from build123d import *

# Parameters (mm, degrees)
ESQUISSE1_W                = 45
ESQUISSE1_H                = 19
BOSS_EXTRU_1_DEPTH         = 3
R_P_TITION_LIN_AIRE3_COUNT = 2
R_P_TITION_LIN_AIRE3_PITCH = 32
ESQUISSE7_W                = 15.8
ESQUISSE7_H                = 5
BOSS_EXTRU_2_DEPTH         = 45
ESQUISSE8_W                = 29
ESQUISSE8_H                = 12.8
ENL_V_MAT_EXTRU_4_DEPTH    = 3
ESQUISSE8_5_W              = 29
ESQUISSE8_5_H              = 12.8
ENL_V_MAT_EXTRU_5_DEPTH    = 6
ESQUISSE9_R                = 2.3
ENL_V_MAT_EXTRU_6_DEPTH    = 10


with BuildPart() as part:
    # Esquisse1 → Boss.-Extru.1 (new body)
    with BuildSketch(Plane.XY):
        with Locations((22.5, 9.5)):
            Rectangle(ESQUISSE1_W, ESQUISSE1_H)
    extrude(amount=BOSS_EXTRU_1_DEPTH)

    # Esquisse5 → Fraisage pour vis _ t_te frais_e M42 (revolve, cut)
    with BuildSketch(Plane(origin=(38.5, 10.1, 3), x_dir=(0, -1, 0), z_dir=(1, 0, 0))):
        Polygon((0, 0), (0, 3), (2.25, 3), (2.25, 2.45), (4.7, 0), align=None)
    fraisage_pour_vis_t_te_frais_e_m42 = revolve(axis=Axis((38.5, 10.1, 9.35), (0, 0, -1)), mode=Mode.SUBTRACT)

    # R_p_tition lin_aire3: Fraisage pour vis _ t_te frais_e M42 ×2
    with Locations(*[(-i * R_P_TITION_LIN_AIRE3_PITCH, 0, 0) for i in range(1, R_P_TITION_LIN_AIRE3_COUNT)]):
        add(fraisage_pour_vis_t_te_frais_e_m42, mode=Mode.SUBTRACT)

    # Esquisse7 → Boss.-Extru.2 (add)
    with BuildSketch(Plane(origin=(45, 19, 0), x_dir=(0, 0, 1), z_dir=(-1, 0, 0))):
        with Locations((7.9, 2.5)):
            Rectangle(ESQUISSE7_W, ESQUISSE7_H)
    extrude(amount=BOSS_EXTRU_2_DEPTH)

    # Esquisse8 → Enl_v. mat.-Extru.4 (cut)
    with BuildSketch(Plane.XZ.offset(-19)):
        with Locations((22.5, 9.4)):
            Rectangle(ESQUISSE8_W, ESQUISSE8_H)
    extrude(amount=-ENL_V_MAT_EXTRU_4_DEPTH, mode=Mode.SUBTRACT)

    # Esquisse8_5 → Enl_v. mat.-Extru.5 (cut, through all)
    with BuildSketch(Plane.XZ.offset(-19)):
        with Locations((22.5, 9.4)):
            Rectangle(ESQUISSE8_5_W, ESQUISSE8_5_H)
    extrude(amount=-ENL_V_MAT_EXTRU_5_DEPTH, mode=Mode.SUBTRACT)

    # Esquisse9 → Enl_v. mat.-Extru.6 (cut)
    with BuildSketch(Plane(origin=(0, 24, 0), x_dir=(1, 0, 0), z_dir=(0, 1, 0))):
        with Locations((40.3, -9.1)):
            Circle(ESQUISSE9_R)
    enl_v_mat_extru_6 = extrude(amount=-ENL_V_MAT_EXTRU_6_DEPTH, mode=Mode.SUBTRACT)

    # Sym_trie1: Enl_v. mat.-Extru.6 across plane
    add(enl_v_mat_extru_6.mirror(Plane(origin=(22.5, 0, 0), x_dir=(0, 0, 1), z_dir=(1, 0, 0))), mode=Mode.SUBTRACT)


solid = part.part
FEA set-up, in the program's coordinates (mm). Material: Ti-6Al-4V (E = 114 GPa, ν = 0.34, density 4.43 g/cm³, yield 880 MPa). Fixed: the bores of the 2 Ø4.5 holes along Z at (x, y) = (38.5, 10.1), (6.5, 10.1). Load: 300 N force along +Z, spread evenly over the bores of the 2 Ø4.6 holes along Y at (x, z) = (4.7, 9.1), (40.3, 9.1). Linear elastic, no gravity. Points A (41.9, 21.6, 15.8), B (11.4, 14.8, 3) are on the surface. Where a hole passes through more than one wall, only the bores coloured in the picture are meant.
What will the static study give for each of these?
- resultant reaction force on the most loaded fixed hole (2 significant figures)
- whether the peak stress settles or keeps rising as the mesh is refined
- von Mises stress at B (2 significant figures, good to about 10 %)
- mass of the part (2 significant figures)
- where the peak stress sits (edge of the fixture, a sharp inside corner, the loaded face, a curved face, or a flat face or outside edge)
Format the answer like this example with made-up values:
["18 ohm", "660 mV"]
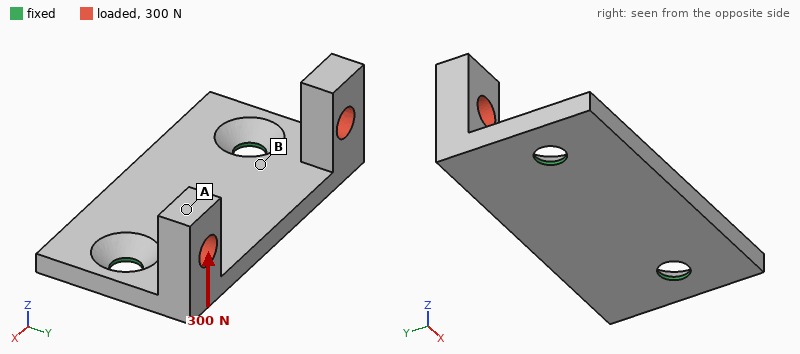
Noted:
["150 N", "keeps rising", "56 MPa", "17 g", "edge of the fixture"]
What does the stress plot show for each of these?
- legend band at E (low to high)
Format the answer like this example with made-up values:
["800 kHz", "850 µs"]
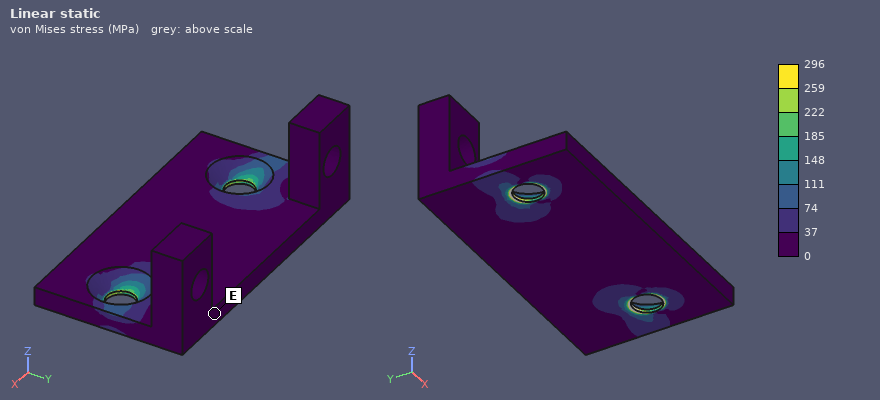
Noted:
["0 to 37 MPa"]
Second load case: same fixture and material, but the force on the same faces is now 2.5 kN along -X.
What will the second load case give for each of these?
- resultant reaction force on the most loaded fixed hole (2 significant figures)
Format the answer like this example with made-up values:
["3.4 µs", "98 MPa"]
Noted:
["1.6 kN"]
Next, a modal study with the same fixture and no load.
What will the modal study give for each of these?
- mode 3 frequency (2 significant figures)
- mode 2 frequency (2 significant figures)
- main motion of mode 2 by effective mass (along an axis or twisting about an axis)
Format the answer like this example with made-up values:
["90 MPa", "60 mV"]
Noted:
["6700 Hz", "4700 Hz", "twisting about Y"]
